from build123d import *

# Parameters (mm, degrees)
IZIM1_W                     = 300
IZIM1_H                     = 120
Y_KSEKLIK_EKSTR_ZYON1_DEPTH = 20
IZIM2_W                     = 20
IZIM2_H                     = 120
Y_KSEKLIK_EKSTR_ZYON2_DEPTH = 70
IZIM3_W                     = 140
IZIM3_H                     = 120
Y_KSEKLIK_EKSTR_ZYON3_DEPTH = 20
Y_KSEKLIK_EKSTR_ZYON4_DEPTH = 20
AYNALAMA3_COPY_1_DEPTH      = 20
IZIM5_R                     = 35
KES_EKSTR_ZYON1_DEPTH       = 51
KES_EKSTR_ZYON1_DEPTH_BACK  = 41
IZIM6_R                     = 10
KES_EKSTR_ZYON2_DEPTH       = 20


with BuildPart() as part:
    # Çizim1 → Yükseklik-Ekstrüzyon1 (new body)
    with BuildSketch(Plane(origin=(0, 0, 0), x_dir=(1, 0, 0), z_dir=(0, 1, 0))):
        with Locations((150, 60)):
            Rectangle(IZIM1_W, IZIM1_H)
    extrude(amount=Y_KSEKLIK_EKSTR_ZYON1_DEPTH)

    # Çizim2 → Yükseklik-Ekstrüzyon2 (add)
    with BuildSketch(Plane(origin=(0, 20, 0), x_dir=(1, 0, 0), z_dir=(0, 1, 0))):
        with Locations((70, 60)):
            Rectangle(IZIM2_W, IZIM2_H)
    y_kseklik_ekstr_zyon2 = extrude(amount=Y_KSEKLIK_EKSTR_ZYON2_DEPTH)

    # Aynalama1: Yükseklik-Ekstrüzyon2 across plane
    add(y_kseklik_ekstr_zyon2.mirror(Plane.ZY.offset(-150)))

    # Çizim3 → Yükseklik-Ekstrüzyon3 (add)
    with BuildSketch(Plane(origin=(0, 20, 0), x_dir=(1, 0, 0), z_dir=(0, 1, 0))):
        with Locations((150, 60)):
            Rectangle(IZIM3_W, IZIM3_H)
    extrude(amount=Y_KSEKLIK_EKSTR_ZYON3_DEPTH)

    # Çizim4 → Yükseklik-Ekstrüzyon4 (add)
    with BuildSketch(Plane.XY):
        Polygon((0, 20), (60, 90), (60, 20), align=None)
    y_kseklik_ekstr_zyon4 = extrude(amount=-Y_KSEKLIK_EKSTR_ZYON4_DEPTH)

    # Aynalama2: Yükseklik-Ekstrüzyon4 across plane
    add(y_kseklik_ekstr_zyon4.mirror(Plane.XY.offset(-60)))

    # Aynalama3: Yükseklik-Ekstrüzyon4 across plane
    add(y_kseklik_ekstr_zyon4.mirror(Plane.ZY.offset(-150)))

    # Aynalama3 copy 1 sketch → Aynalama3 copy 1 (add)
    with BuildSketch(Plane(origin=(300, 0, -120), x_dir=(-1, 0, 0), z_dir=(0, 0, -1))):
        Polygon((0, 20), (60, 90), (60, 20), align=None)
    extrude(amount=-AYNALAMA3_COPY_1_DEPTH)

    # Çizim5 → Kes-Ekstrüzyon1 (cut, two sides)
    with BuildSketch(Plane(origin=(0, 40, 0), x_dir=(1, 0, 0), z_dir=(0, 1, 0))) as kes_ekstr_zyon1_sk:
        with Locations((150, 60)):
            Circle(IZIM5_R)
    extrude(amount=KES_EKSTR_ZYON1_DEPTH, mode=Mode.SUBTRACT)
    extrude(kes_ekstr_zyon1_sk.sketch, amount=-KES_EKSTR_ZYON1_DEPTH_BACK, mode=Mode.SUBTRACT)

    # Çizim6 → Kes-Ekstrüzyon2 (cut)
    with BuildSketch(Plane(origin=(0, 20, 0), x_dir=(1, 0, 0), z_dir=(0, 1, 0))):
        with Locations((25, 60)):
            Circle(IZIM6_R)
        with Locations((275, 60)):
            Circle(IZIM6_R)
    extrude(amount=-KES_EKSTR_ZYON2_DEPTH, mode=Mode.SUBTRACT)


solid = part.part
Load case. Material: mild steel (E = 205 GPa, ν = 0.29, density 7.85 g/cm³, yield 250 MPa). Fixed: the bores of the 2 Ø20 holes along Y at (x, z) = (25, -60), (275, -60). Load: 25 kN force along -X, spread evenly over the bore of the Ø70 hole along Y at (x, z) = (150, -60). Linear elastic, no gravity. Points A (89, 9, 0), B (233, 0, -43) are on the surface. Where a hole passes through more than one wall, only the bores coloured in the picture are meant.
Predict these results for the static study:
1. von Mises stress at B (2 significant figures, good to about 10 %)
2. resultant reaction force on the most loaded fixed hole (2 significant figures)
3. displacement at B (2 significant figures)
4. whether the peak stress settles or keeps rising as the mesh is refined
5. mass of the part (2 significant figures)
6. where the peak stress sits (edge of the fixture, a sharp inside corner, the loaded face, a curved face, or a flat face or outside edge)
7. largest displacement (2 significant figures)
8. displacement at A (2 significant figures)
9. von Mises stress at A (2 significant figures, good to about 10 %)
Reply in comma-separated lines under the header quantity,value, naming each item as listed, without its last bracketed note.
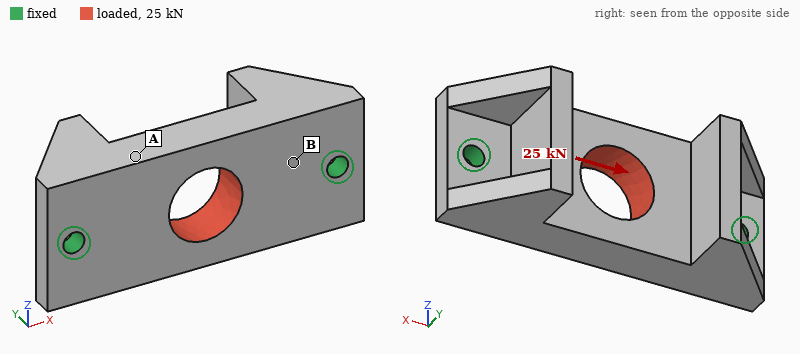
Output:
quantity,value
von Mises stress at B,6.5 MPa
resultant reaction force on the most loaded fixed hole,13 kN
displacement at B,1.7 µm
whether the peak stress settles or keeps rising as the mesh is refined,keeps rising
mass of the part,11 kg
where the peak stress sits,edge of the fixture
largest displacement,3.7 µm
displacement at A,2.7 µm
von Mises stress at A,2.6 MPa
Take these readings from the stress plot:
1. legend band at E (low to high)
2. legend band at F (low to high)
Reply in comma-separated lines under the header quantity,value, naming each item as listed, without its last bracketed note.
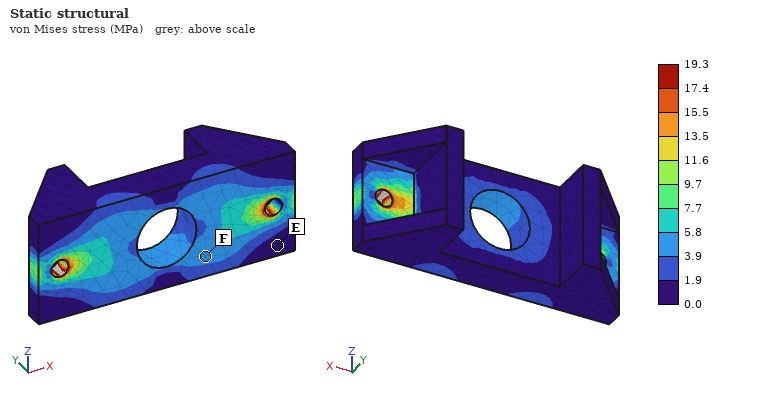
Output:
quantity,value
legend band at E,0.0 to 1.9 MPa
legend band at F,3.9 to 5.8 MPa
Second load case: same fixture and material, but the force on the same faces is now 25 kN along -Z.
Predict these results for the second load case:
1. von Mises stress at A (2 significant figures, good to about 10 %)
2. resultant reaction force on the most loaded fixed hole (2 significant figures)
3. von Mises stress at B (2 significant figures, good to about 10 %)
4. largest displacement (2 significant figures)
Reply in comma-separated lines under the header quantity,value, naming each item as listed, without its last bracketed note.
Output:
quantity,value
von Mises stress at A,8.3 MPa
resultant reaction force on the most loaded fixed hole,13 kN
von Mises stress at B,6.2 MPa
largest displacement,23 µm
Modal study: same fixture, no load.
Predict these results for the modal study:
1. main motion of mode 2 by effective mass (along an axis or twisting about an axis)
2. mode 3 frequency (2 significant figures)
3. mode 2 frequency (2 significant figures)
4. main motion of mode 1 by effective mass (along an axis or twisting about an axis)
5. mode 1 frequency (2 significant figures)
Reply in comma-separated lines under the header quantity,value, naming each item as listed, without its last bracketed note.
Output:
quantity,value
main motion of mode 2 by effective mass,along Y
mode 3 frequency,2500 Hz
mode 2 frequency,1600 Hz
main motion of mode 1 by effective mass,along Z
mode 1 frequency,1300 Hz
